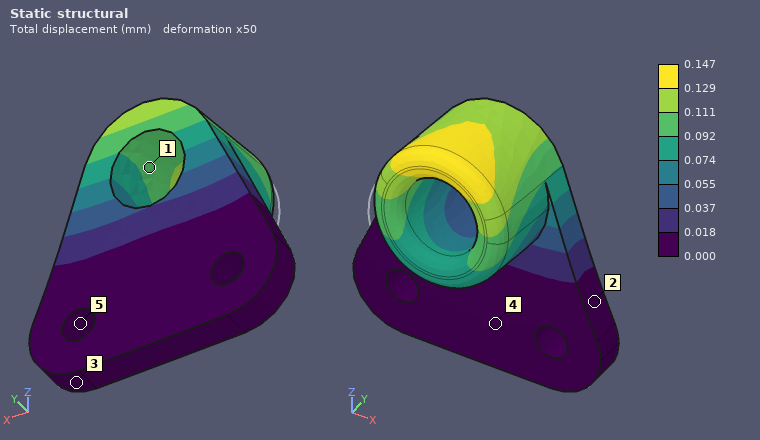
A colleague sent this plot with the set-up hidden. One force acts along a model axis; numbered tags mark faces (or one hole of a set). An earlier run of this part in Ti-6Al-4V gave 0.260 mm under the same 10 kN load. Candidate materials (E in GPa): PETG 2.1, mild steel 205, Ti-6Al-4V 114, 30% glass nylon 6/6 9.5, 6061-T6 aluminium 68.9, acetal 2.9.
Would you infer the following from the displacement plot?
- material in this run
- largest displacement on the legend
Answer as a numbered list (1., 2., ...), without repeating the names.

1. mild steel
2. 0.147 mm
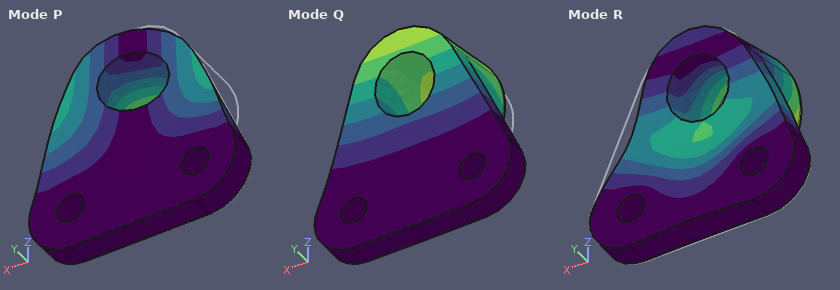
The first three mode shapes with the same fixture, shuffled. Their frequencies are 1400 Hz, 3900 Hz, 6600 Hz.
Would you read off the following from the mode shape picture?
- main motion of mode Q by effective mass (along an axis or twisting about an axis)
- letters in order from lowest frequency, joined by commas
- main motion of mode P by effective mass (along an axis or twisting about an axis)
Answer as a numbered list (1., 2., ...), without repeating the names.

1. along Y
2. Q, P, R
3. along X
